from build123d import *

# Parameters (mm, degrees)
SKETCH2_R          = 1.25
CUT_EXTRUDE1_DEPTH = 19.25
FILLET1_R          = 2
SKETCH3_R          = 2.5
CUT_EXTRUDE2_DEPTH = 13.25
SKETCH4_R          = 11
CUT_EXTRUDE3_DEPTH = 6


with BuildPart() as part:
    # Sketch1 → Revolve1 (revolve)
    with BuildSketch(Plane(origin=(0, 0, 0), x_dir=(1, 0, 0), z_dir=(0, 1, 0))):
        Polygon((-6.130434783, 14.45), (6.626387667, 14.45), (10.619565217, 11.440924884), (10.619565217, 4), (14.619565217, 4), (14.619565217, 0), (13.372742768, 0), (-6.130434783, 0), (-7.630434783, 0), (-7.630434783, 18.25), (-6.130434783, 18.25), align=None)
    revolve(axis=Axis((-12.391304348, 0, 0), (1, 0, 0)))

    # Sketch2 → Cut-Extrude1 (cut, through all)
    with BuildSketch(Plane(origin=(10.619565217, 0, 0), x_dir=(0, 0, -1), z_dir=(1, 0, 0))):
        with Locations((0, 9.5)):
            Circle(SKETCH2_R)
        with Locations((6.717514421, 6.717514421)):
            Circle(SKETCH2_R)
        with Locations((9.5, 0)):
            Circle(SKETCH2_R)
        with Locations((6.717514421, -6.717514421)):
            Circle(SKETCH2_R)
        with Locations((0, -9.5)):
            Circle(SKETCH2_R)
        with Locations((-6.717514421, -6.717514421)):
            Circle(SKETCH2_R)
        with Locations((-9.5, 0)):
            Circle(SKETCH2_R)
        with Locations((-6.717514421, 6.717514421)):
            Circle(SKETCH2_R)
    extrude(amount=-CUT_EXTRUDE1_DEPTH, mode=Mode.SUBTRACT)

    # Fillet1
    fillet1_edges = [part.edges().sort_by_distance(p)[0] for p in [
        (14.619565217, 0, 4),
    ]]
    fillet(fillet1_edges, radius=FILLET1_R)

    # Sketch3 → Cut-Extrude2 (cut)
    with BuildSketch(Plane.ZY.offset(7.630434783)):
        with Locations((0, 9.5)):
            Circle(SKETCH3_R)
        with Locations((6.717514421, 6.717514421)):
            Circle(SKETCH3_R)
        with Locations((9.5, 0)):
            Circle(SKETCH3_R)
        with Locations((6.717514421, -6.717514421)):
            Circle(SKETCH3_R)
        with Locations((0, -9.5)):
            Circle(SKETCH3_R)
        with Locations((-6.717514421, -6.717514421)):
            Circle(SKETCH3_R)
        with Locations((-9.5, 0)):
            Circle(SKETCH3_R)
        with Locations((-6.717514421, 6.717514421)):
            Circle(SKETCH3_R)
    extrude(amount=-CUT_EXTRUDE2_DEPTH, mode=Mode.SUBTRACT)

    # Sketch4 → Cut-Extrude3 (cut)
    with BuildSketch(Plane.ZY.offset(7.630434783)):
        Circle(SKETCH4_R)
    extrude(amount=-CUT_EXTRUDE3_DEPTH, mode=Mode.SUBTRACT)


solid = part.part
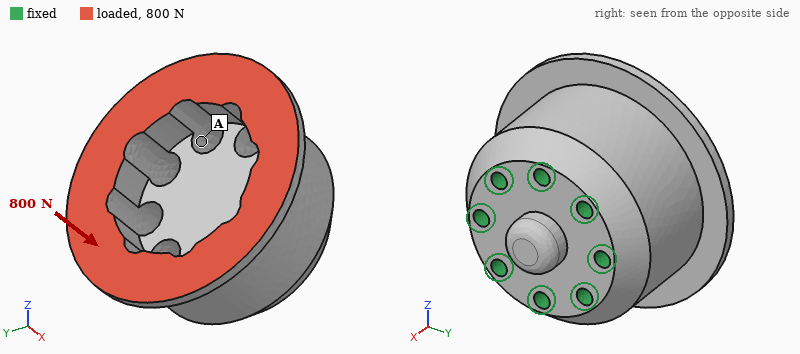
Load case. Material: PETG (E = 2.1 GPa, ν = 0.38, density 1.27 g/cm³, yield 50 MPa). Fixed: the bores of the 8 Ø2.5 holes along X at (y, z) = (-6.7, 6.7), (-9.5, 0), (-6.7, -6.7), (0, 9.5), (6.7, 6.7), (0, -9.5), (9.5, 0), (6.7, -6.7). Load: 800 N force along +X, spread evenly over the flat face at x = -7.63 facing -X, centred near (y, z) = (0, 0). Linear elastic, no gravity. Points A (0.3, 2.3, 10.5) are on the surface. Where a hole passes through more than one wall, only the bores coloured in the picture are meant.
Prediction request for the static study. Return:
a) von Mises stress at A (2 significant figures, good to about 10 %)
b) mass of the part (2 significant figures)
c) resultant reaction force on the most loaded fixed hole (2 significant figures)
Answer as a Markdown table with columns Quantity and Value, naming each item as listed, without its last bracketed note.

| Quantity | Value |
|---|---|
| von Mises stress at A | 3.1 MPa |
| mass of the part | 11 g |
| resultant reaction force on the most loaded fixed hole | 100 N |
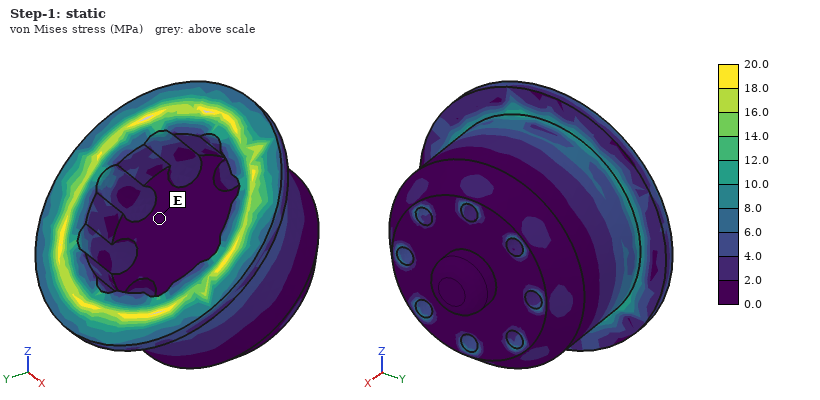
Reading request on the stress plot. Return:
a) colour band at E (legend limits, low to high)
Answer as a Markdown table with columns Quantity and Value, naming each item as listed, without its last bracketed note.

| Quantity | Value |
|---|---|
| colour band at E | 0.0 to 2.0 MPa |
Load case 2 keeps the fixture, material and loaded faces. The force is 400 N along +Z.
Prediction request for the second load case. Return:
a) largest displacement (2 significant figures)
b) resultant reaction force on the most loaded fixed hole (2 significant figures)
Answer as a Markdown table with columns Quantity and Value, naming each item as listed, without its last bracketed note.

| Quantity | Value |
|---|---|
| largest displacement | 0.15 mm |
| resultant reaction force on the most loaded fixed hole | 140 N |
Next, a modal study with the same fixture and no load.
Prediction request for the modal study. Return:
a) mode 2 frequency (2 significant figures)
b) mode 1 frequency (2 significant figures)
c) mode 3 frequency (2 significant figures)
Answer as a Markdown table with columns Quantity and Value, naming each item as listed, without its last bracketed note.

| Quantity | Value |
|---|---|
| mode 2 frequency | 6900 Hz |
| mode 1 frequency | 6900 Hz |
| mode 3 frequency | 7800 Hz |
